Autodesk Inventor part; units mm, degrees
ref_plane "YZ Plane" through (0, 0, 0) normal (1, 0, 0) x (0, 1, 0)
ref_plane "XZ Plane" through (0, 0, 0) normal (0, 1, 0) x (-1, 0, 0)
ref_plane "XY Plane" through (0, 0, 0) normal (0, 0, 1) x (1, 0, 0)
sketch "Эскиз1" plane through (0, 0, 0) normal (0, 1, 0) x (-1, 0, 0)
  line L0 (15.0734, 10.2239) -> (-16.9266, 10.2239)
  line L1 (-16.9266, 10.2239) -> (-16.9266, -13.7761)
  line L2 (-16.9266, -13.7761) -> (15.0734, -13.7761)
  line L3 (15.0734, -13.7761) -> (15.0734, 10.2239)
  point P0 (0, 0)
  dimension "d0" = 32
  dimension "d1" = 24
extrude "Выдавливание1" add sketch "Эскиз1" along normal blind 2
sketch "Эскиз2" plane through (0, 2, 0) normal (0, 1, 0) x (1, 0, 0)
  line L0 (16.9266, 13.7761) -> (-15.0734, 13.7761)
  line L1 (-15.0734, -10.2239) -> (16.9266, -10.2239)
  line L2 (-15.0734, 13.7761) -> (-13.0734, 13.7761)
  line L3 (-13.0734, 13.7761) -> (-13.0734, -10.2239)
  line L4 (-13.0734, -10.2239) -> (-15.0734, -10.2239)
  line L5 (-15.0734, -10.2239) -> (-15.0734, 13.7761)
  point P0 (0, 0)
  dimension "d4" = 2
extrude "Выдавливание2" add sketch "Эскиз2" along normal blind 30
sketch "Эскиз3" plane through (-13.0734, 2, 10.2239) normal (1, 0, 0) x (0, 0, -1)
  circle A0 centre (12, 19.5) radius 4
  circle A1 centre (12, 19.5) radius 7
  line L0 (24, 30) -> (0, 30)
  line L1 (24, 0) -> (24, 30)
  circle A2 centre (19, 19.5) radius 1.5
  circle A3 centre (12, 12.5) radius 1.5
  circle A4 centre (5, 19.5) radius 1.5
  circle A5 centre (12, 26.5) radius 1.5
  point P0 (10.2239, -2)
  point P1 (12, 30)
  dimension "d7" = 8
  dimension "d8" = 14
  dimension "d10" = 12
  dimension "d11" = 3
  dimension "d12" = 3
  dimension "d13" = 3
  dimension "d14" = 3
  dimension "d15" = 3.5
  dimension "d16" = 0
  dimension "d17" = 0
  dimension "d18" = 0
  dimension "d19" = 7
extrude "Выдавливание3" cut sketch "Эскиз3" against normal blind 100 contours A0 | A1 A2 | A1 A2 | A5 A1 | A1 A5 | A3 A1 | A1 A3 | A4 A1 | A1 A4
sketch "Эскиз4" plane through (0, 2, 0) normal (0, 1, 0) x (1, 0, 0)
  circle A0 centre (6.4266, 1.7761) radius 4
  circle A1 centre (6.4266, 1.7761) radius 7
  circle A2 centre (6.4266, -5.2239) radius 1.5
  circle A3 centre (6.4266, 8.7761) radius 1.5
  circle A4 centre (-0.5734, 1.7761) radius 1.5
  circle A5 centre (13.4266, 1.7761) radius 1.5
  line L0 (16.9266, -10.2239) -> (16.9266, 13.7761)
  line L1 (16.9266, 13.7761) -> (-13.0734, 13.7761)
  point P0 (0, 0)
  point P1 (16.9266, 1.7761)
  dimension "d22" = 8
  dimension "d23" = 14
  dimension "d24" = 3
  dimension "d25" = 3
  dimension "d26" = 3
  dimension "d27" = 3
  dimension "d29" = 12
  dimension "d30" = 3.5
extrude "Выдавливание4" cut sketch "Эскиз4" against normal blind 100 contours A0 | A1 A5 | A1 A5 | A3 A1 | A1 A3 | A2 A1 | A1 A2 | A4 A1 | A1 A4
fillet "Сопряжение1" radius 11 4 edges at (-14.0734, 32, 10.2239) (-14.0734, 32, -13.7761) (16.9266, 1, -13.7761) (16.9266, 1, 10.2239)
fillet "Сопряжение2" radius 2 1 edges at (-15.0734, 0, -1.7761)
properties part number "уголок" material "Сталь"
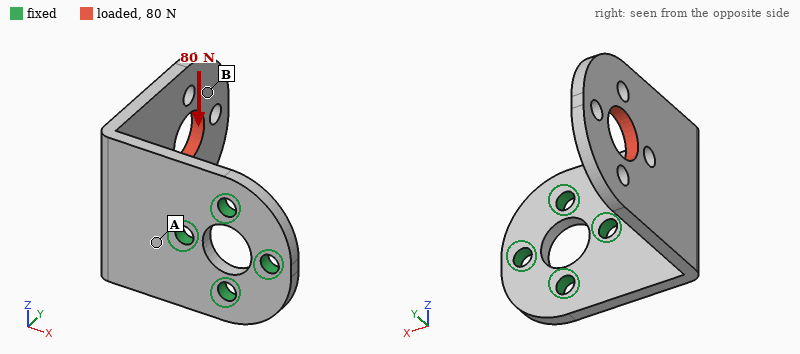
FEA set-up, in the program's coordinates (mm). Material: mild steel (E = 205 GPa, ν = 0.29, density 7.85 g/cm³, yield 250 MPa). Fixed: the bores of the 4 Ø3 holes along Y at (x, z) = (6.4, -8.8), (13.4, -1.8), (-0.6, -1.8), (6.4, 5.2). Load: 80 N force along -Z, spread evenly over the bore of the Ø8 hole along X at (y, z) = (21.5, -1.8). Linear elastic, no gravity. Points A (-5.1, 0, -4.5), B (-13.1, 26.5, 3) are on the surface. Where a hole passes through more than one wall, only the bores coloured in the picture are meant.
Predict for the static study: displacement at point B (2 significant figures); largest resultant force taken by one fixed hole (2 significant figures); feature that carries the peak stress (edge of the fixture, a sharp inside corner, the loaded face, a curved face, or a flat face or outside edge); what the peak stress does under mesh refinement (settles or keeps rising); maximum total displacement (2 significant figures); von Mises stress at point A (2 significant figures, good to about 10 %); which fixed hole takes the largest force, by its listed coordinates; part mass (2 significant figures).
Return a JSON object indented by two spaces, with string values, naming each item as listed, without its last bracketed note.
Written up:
{
  "displacement at point B": "0.094 mm",
  "largest resultant force taken by one fixed hole": "91 N",
  "feature that carries the peak stress": "edge of the fixture",
  "what the peak stress does under mesh refinement": "keeps rising",
  "maximum total displacement": "0.11 mm",
  "von Mises stress at point A": "65 MPa",
  "which fixed hole takes the largest force, by its listed coordinates": "(-0.6, -1.8)",
  "part mass": "19 g"
}
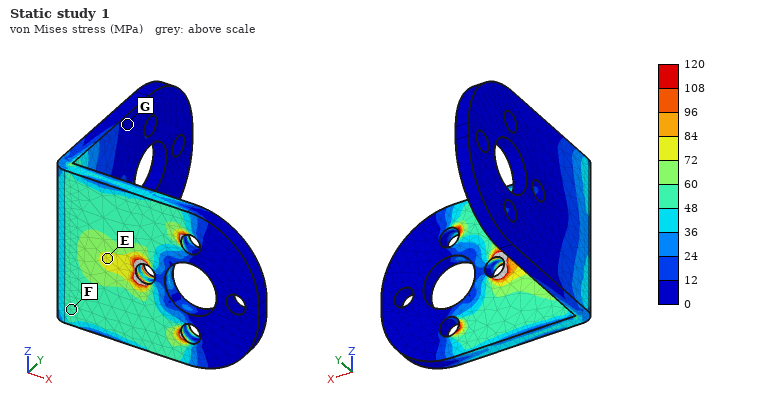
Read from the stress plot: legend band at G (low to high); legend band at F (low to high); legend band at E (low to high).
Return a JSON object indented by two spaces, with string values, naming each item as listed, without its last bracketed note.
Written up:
{
  "legend band at G": "0 to 12 MPa",
  "legend band at F": "48 to 60 MPa",
  "legend band at E": "72 to 84 MPa"
}
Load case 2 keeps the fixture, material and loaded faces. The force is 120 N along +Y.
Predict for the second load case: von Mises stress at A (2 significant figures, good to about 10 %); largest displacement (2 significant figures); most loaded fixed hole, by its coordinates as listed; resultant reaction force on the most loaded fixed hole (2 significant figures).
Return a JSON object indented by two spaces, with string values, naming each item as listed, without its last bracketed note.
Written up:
{
  "von Mises stress at A": "73 MPa",
  "largest displacement": "0.11 mm",
  "most loaded fixed hole, by its coordinates as listed": "(-0.6, -1.8)",
  "resultant reaction force on the most loaded fixed hole": "190 N"
}
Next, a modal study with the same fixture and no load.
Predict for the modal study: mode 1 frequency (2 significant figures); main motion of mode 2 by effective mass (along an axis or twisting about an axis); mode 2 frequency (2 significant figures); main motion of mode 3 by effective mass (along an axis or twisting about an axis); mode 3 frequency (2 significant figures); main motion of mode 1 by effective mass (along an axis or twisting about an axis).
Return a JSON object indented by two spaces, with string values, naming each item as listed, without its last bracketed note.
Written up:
{
  "mode 1 frequency": "1200 Hz",
  "main motion of mode 2 by effective mass": "along Z",
  "mode 2 frequency": "1900 Hz",
  "main motion of mode 3 by effective mass": "along Y",
  "mode 3 frequency": "4100 Hz",
  "main motion of mode 1 by effective mass": "along X"
}
